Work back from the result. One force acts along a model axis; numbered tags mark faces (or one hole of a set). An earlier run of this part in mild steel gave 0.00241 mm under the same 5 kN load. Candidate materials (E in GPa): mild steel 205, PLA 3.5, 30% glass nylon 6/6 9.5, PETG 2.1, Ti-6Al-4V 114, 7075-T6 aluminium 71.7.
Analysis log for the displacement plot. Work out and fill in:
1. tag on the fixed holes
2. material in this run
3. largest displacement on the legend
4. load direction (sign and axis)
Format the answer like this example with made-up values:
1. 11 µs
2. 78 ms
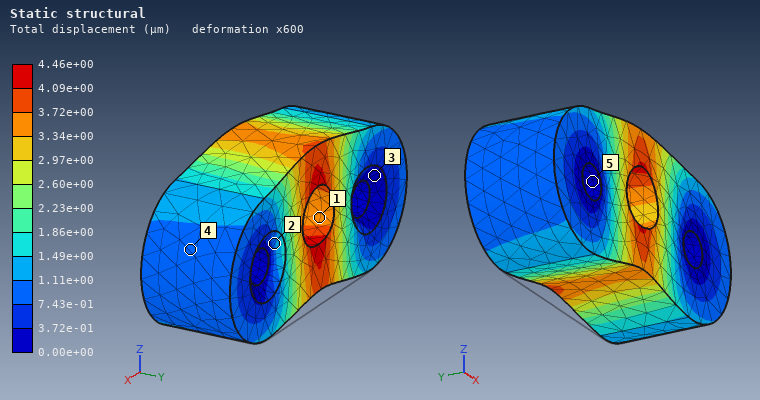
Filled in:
1. 5
2. Ti-6Al-4V
3. 4.46e+00 µm
4. +Z
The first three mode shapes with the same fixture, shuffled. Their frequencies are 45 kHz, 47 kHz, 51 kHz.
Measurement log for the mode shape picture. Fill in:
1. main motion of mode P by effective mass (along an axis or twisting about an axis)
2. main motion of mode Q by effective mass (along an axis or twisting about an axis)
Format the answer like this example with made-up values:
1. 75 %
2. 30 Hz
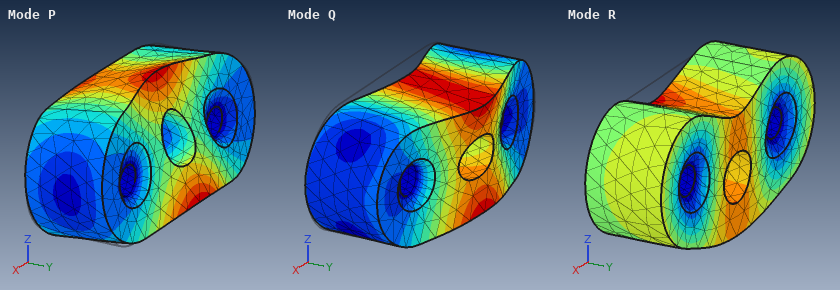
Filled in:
1. twisting about X
2. along Y
